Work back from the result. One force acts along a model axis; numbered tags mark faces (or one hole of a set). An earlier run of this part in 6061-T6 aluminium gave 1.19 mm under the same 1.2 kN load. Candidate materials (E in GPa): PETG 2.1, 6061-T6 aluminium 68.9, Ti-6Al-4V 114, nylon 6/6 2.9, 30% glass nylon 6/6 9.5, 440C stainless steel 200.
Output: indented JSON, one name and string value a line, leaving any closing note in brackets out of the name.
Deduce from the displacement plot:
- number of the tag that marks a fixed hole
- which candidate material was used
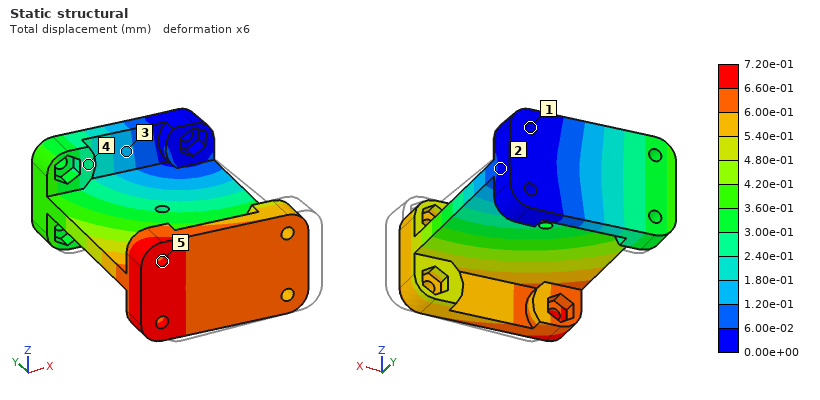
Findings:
{
  "number of the tag that marks a fixed hole": "1",
  "which candidate material was used": "Ti-6Al-4V"
}
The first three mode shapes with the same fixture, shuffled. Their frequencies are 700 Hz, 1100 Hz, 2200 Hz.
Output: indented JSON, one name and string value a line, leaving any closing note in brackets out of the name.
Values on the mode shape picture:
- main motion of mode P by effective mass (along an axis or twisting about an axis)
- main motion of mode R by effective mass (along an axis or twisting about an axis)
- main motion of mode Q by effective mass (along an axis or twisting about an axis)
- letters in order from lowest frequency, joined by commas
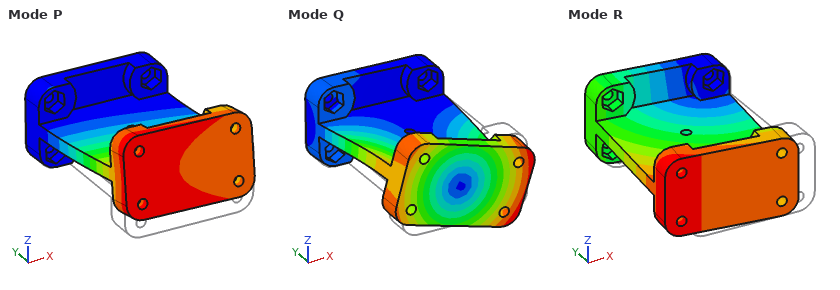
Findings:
{
  "main motion of mode P by effective mass": "along Z",
  "main motion of mode R by effective mass": "along X",
  "main motion of mode Q by effective mass": "twisting about Y",
  "letters in order from lowest frequency, joined by commas": "P, R, Q"
}
